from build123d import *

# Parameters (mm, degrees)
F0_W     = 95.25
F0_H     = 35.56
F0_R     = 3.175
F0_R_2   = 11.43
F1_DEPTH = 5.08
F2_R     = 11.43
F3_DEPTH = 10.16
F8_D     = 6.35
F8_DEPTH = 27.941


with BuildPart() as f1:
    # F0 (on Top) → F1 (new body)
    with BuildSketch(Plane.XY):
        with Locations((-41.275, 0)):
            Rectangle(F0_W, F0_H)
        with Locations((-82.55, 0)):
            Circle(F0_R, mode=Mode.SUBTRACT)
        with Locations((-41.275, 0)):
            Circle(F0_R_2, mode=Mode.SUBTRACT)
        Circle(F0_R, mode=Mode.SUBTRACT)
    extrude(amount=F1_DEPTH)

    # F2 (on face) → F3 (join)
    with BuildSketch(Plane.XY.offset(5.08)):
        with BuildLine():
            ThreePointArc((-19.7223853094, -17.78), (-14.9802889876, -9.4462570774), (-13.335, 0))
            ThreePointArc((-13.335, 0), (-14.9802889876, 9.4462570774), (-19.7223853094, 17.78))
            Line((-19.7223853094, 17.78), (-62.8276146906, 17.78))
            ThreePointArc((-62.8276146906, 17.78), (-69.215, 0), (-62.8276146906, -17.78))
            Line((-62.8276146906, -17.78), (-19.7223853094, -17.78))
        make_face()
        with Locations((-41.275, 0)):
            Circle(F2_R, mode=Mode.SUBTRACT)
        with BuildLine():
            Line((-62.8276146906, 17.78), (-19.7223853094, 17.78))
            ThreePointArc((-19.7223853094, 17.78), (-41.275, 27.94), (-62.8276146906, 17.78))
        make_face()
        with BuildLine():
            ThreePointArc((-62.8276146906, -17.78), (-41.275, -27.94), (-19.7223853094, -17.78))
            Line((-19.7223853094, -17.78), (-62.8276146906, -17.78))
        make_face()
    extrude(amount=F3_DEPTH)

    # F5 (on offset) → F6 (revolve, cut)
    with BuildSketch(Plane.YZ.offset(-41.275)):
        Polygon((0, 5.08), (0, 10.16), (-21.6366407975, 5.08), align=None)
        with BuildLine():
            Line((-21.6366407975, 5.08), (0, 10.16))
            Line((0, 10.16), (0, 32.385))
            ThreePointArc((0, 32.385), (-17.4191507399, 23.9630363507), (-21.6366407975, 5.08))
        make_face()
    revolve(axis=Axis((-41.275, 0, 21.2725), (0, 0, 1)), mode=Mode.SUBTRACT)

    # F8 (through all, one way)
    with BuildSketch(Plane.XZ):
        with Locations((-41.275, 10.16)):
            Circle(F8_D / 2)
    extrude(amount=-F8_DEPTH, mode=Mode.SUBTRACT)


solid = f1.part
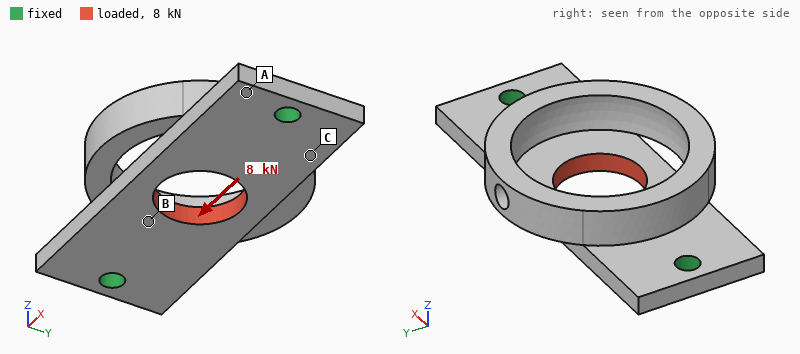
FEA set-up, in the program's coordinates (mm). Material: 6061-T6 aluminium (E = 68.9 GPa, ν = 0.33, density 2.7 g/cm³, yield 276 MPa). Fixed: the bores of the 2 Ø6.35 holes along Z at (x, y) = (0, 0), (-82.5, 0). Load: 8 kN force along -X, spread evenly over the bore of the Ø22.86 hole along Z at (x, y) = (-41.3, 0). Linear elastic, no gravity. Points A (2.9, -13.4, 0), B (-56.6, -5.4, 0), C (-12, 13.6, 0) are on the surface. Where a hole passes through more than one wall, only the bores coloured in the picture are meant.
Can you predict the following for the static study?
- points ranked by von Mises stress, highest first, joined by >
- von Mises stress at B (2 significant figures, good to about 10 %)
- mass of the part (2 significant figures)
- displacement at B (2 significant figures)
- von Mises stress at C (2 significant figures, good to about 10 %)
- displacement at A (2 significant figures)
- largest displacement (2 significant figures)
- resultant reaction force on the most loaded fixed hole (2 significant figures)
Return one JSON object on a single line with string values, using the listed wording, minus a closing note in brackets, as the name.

{"points ranked by von Mises stress, highest first, joined by >": "B > C > A", "von Mises stress at B": "29 MPa", "mass of the part": "65 g", "displacement at B": "13 µm", "von Mises stress at C": "17 MPa", "displacement at A": "7.5 µm", "largest displacement": "18 µm", "resultant reaction force on the most loaded fixed hole": "4.0 kN"}
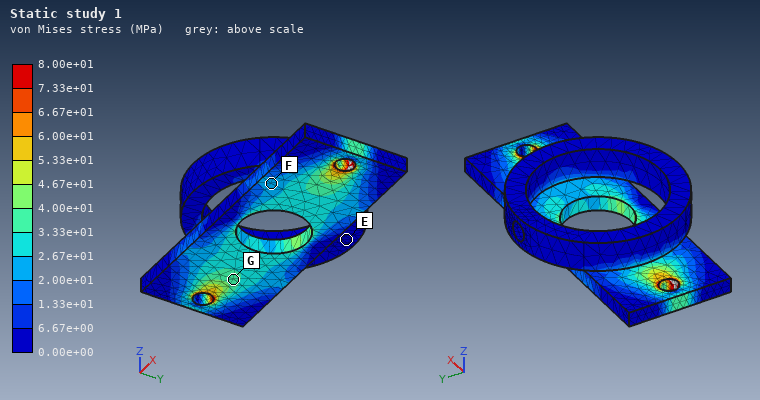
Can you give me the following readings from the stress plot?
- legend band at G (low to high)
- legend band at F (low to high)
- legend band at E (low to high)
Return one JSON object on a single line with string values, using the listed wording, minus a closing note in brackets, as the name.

{"legend band at G": "3.33e+01 to 4.00e+01 MPa", "legend band at F": "2.00e+01 to 2.67e+01 MPa", "legend band at E": "0.00e+00 to 6.67e+00 MPa"}
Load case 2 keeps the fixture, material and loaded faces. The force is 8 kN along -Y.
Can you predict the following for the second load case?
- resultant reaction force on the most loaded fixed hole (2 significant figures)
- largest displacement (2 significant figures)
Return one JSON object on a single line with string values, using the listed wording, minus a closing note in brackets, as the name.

{"resultant reaction force on the most loaded fixed hole": "4.0 kN", "largest displacement": "77 µm"}
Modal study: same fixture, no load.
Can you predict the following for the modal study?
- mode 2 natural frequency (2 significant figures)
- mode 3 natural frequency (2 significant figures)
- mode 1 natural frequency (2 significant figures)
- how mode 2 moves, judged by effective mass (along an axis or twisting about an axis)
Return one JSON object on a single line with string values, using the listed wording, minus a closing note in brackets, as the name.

{"mode 2 natural frequency": "3800 Hz", "mode 3 natural frequency": "8800 Hz", "mode 1 natural frequency": "3100 Hz", "how mode 2 moves, judged by effective mass": "along Z"}
